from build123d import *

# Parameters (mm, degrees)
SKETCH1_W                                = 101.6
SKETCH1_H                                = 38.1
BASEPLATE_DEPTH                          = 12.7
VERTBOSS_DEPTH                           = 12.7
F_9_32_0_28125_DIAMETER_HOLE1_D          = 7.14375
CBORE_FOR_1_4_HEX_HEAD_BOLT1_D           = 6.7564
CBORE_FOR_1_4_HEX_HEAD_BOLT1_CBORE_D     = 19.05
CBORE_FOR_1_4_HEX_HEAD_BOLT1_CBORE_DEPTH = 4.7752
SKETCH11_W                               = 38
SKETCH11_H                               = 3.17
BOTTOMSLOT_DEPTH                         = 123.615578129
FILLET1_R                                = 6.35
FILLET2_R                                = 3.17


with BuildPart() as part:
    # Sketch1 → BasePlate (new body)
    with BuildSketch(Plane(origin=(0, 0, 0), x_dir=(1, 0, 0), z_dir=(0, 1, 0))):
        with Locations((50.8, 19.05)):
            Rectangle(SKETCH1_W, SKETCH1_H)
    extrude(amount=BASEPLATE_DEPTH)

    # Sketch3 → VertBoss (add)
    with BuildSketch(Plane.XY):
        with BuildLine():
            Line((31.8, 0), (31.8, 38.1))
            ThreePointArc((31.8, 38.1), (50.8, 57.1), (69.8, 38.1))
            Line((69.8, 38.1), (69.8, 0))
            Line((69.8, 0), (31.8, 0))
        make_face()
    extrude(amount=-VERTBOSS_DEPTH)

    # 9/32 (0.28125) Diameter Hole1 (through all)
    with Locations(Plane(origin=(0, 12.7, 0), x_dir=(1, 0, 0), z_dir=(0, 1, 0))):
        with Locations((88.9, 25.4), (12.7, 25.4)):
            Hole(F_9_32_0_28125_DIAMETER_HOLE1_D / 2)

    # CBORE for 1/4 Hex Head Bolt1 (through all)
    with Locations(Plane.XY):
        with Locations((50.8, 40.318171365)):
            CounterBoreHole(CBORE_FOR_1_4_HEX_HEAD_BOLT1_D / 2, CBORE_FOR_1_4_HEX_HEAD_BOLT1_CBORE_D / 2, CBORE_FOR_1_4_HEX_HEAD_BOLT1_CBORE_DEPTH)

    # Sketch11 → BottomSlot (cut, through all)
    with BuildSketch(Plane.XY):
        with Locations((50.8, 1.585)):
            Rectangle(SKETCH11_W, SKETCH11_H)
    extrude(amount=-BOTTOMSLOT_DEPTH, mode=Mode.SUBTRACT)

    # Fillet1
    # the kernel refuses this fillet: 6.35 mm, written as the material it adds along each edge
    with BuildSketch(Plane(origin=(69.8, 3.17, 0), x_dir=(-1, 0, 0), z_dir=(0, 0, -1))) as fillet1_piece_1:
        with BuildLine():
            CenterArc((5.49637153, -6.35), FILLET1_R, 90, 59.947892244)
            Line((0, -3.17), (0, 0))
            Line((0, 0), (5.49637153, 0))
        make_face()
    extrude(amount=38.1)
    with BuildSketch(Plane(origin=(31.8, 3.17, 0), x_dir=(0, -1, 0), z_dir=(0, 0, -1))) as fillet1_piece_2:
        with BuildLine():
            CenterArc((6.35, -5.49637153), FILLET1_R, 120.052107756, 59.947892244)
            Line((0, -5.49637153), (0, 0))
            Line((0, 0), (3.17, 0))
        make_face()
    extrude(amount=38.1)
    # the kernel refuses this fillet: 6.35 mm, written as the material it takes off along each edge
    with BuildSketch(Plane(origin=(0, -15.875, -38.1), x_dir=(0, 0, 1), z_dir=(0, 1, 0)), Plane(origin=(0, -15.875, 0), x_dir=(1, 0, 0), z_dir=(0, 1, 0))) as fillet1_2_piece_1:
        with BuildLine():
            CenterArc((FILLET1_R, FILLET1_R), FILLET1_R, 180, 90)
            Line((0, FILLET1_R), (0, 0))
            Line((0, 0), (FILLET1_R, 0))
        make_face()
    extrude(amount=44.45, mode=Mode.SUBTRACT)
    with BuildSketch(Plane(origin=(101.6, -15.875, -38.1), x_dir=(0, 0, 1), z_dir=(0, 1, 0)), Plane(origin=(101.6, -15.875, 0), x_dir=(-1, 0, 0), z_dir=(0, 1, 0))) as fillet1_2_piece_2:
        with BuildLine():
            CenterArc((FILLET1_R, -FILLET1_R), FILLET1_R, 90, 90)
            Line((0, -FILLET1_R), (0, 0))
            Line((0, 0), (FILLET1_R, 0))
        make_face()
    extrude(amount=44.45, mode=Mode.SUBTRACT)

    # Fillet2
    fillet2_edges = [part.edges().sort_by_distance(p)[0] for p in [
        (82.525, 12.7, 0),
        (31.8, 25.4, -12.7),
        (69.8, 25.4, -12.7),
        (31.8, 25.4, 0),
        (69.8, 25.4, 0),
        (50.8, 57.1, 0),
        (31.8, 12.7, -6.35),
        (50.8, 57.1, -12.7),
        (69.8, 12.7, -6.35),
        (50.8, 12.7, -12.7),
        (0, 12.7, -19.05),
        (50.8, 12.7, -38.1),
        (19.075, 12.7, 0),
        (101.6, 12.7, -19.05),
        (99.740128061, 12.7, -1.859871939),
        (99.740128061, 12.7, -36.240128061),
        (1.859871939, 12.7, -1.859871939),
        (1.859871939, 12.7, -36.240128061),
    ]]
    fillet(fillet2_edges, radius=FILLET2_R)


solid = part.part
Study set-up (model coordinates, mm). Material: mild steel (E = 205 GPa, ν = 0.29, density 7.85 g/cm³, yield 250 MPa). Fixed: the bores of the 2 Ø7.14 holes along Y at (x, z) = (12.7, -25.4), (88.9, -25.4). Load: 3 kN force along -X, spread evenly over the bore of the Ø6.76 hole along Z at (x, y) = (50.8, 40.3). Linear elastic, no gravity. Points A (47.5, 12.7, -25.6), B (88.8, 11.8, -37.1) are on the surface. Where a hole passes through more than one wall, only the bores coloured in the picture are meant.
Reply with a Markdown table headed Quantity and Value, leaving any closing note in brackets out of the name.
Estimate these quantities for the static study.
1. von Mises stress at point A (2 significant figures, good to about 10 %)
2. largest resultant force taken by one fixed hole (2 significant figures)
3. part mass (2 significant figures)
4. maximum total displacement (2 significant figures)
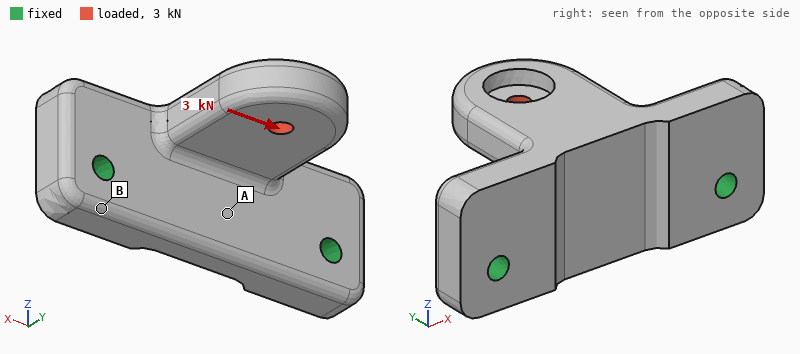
| Quantity | Value |
|---|---|
| von Mises stress at point A | 17 MPa |
| largest resultant force taken by one fixed hole | 2.3 kN |
| part mass | 470 g |
| maximum total displacement | 24 µm |
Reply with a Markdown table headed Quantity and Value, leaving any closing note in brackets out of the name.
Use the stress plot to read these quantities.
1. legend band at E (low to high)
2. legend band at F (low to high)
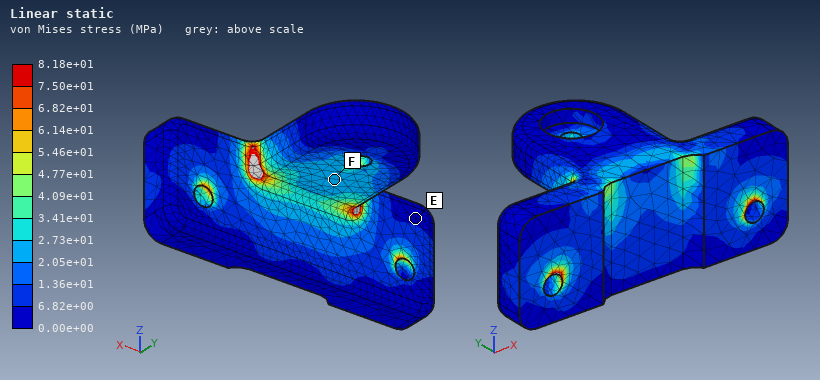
| Quantity | Value |
|---|---|
| legend band at E | 0.00e+00 to 6.82e+00 MPa |
| legend band at F | 2.05e+01 to 2.73e+01 MPa |
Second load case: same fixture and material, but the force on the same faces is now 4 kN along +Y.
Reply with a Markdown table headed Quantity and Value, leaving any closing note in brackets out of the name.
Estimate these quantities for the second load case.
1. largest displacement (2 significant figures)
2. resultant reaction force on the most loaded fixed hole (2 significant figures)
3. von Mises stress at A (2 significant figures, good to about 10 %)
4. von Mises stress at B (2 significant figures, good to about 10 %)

| Quantity | Value |
|---|---|
| largest displacement | 24 µm |
| resultant reaction force on the most loaded fixed hole | 2.1 kN |
| von Mises stress at A | 13 MPa |
| von Mises stress at B | 8.1 MPa |
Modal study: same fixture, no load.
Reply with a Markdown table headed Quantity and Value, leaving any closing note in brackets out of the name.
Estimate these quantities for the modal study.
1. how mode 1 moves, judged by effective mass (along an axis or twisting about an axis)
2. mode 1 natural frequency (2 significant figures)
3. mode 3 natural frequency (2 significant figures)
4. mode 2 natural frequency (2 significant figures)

| Quantity | Value |
|---|---|
| how mode 1 moves, judged by effective mass | along Z |
| mode 1 natural frequency | 3100 Hz |
| mode 3 natural frequency | 6600 Hz |
| mode 2 natural frequency | 6400 Hz |
